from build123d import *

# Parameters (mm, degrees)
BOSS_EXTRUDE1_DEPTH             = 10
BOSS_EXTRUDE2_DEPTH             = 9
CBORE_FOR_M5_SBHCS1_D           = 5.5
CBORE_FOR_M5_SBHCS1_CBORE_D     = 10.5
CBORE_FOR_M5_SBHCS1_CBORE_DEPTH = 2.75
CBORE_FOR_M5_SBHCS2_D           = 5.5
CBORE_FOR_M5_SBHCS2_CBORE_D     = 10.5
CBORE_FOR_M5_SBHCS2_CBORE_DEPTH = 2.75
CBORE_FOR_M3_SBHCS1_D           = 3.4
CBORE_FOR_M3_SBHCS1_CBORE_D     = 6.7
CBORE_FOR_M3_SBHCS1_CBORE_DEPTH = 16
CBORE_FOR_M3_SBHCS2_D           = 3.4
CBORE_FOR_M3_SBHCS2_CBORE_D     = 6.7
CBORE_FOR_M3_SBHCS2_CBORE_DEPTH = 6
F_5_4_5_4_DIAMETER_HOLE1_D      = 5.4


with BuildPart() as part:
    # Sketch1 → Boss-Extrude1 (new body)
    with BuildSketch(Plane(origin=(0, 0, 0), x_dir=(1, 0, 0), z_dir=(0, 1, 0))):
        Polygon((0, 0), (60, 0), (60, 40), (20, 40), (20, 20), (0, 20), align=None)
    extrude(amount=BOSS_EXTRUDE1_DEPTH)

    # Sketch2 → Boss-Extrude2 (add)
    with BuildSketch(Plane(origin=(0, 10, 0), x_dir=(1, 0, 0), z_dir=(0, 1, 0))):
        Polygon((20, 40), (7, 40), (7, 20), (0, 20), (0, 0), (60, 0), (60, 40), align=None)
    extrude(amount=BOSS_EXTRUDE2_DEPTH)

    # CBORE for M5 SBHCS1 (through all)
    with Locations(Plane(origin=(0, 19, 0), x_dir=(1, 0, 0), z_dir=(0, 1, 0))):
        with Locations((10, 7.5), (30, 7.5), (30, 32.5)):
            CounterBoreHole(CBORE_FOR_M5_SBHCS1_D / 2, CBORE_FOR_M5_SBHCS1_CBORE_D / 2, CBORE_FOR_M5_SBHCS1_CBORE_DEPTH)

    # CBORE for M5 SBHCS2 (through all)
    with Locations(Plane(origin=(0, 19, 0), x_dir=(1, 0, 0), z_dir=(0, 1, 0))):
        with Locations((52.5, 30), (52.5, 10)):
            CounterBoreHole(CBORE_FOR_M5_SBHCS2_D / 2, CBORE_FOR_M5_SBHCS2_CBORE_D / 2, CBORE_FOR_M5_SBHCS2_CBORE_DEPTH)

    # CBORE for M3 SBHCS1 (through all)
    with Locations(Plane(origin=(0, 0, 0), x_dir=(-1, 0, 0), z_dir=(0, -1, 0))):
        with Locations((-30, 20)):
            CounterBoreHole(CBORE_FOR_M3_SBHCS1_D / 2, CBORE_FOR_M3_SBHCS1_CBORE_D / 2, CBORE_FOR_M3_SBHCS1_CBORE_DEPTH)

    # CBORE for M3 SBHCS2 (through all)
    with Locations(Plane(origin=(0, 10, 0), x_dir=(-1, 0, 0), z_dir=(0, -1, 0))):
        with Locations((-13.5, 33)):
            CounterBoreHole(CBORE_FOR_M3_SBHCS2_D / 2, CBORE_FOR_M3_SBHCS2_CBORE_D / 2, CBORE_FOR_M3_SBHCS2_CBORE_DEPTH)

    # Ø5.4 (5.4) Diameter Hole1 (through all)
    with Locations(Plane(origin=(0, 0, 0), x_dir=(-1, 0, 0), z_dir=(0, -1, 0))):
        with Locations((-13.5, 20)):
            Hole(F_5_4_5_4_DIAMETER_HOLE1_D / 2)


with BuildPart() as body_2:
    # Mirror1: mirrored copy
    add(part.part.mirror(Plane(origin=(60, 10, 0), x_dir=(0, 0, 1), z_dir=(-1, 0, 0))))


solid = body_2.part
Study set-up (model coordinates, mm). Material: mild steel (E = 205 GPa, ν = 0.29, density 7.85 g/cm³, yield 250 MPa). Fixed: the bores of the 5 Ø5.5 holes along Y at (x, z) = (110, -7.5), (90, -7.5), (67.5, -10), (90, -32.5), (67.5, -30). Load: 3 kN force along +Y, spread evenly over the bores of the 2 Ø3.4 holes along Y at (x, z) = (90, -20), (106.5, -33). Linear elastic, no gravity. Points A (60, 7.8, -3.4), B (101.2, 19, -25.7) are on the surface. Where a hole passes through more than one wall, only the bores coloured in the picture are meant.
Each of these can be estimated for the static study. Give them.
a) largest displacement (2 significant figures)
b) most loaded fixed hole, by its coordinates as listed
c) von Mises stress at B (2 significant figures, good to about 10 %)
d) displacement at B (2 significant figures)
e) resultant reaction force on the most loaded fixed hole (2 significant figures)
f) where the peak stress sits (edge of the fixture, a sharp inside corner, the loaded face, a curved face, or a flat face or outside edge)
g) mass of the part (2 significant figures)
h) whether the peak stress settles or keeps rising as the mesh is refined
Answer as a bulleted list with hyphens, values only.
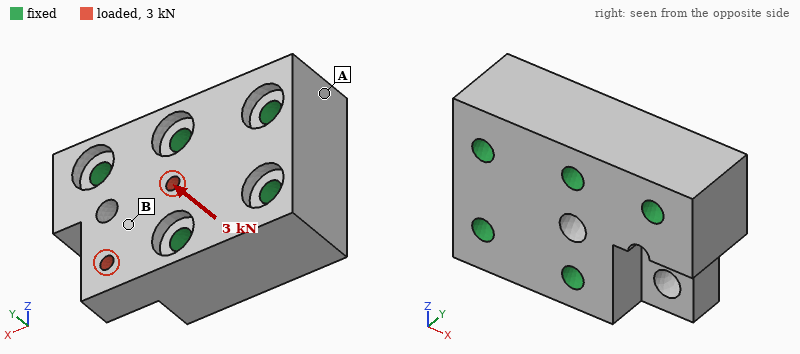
- 7.4 µm
- (90, -32.5)
- 27 MPa
- 1.7 µm
- 1.9 kN
- a sharp inside corner
- 280 g
- keeps rising
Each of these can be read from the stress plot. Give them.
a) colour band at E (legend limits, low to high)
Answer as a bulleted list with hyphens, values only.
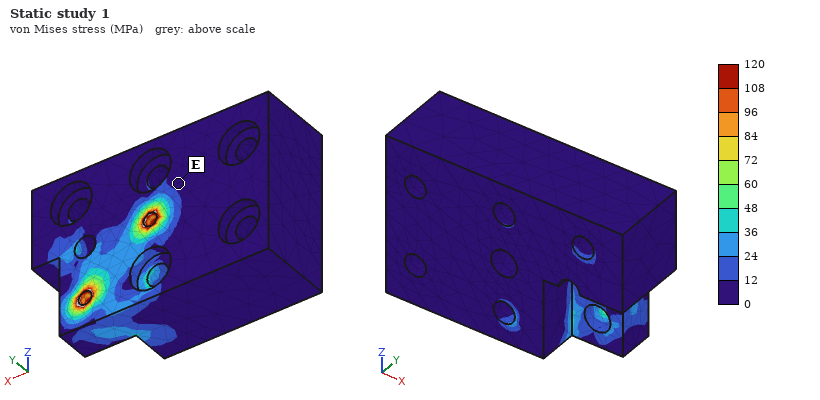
- 0 to 12 MPa
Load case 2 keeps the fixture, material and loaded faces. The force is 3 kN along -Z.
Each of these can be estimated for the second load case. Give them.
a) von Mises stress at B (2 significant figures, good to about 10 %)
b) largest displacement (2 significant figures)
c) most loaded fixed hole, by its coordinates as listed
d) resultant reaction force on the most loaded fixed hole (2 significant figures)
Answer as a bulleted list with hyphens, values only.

- 17 MPa
- 3.3 µm
- (90, -32.5)
- 1.2 kN
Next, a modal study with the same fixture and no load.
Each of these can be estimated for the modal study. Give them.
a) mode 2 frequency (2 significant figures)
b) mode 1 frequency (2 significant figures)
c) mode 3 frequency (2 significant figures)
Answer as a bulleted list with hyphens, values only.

- 41 kHz
- 25 kHz
- 46 kHz
